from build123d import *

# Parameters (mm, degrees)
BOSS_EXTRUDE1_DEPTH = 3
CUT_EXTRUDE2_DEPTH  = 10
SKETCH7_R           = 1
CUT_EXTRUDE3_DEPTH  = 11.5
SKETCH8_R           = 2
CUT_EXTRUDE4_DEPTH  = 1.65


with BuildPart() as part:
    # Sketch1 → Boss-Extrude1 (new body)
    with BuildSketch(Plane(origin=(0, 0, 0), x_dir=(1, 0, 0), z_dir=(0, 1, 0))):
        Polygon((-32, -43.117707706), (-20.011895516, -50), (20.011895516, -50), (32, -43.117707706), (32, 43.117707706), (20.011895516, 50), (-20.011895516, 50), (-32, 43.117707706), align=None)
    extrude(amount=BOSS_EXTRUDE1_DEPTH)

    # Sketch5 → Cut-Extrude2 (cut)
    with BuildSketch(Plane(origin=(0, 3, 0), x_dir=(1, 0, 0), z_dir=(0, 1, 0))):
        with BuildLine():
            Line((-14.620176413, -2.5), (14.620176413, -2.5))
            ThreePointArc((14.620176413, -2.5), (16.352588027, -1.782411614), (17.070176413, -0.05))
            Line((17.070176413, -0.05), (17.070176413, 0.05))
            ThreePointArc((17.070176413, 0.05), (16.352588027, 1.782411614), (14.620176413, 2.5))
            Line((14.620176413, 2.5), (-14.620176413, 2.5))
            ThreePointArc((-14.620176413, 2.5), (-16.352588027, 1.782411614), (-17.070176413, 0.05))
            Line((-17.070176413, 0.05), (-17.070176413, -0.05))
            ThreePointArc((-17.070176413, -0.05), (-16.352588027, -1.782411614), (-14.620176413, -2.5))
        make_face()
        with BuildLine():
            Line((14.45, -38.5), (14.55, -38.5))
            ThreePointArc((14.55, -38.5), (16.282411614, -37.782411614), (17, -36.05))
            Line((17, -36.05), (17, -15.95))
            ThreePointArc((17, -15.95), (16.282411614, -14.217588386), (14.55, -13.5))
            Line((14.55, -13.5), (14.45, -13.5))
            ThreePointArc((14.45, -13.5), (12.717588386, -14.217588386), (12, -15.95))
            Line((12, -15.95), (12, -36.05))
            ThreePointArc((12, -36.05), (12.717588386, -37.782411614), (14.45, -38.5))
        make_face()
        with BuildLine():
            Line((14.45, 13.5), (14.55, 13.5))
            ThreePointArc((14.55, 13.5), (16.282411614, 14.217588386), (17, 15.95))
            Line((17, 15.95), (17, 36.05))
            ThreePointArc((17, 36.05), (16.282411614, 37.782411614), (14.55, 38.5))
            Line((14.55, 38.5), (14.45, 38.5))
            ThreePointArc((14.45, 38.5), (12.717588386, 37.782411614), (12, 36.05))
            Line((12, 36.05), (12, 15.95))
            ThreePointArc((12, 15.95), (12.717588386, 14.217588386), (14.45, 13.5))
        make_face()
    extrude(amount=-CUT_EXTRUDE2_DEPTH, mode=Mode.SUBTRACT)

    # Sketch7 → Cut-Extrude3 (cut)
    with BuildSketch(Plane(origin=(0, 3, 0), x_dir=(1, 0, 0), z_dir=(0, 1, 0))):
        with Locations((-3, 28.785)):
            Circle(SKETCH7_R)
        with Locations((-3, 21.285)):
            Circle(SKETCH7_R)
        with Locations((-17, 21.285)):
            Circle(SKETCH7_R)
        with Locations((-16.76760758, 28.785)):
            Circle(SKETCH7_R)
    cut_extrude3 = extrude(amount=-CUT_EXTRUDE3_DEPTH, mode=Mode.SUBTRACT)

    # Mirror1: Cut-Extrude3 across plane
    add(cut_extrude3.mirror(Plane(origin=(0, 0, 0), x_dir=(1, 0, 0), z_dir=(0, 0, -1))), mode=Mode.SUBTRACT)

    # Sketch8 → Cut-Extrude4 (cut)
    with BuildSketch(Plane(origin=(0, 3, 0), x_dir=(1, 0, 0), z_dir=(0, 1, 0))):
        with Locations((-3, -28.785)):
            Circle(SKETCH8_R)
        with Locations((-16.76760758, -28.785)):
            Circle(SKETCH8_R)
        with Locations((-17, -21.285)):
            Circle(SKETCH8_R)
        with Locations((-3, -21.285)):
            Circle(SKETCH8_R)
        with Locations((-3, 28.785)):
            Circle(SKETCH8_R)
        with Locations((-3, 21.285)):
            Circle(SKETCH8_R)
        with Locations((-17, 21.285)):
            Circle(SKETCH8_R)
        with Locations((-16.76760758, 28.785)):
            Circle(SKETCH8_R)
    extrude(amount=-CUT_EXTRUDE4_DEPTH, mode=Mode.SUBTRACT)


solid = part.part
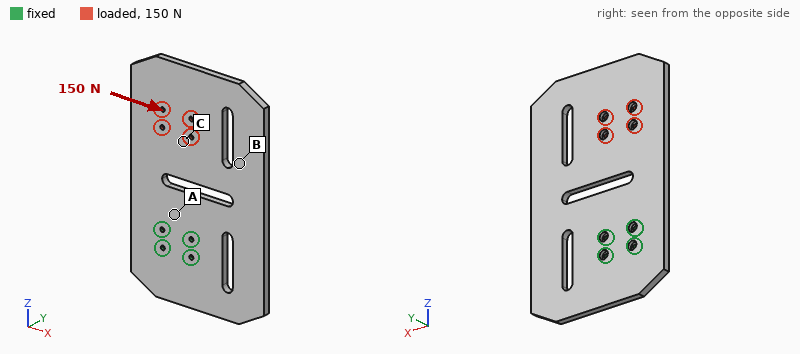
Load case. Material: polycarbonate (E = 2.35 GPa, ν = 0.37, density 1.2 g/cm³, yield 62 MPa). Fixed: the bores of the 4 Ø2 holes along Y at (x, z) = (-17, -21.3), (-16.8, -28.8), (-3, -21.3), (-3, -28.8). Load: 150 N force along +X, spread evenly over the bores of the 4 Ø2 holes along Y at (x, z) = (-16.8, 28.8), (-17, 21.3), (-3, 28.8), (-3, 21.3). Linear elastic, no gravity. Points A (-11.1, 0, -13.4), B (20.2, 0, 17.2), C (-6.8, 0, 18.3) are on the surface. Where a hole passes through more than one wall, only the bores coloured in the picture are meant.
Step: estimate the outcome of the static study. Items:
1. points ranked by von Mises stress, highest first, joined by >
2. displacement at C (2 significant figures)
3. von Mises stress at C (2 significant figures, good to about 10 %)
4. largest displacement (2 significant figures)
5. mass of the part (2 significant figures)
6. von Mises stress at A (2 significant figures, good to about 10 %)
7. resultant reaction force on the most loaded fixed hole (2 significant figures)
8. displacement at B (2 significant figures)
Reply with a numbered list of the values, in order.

1. A > C > B
2. 0.41 mm
3. 3.8 MPa
4. 0.88 mm
5. 21 g
6. 8.2 MPa
7. 270 N
8. 0.54 mm
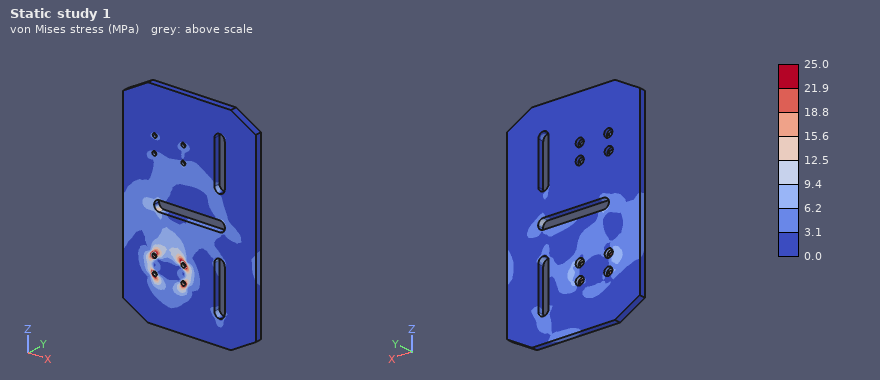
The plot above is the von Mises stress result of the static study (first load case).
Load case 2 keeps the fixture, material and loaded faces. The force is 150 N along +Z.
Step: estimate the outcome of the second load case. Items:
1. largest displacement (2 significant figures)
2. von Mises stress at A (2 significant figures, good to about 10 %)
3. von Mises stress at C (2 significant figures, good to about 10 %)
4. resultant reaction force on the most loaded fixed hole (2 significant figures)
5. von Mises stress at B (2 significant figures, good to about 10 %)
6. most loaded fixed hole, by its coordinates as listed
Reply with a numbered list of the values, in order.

1. 1.3 mm
2. 2.2 MPa
3. 1.9 MPa
4. 51 N
5. 1.6 MPa
6. (-17, -21.3)
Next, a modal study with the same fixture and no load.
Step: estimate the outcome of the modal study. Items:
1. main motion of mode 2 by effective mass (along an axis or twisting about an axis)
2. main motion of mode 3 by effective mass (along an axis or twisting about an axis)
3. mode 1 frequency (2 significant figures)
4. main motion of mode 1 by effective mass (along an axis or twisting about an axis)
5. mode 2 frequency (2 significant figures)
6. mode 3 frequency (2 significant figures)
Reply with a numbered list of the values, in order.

1. twisting about Z
2. along Y
3. 100 Hz
4. along Y
5. 260 Hz
6. 500 Hz
